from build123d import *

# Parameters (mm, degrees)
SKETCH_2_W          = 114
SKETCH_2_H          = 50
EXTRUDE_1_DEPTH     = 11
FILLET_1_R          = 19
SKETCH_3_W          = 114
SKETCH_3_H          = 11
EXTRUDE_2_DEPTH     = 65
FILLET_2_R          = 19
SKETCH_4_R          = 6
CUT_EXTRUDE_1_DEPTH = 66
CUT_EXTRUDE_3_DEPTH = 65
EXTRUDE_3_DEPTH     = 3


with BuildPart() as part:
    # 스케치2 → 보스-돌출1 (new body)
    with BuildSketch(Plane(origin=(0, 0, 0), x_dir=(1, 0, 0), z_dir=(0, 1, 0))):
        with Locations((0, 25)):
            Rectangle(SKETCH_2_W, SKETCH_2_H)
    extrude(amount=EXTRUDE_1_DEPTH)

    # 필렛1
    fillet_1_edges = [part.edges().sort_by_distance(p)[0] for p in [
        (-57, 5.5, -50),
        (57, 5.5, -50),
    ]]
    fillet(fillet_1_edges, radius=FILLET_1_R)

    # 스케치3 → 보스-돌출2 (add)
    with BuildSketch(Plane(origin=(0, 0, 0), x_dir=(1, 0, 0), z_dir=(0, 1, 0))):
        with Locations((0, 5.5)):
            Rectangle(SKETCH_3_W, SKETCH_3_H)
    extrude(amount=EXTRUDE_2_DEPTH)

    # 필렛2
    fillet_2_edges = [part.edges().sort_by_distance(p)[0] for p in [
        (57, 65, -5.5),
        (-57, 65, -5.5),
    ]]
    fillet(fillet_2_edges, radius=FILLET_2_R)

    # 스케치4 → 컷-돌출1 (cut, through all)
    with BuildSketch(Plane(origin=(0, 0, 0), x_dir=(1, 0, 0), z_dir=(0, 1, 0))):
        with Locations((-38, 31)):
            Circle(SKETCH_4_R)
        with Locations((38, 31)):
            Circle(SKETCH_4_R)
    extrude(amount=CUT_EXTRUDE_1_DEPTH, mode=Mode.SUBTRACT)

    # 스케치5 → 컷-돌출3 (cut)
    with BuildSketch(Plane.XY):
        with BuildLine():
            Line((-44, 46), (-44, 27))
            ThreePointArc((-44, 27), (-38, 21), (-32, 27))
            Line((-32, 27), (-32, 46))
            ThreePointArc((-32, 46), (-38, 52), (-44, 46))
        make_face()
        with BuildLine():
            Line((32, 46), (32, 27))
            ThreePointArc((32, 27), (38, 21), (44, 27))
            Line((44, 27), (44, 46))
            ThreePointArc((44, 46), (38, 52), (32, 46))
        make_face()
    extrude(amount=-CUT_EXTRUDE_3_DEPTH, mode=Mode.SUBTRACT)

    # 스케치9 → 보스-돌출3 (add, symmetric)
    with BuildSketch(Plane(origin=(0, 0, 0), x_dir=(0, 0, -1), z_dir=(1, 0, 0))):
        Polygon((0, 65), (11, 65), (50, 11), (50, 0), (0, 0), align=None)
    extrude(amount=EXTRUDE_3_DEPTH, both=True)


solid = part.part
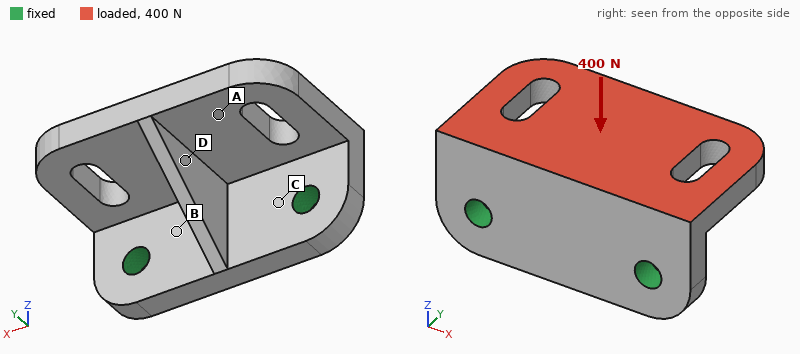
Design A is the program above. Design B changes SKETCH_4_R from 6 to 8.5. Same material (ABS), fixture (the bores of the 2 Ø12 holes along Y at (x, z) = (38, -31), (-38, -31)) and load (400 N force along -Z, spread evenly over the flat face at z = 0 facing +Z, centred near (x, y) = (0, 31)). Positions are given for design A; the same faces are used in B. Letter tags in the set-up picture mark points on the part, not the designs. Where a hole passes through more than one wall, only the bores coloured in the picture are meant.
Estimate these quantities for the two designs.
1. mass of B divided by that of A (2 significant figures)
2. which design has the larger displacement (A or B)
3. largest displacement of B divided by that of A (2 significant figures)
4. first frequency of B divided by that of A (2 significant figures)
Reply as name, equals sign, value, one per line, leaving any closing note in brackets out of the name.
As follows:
mass of B divided by that of A = 0.98
which design has the larger displacement = A
largest displacement of B divided by that of A = 0.83
first frequency of B divided by that of A = 1.1
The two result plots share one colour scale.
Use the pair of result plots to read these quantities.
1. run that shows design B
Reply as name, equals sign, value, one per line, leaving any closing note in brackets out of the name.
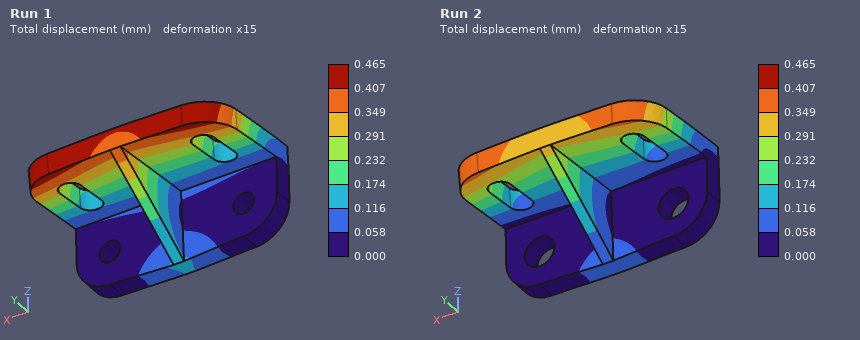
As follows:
run that shows design B = Run 2
